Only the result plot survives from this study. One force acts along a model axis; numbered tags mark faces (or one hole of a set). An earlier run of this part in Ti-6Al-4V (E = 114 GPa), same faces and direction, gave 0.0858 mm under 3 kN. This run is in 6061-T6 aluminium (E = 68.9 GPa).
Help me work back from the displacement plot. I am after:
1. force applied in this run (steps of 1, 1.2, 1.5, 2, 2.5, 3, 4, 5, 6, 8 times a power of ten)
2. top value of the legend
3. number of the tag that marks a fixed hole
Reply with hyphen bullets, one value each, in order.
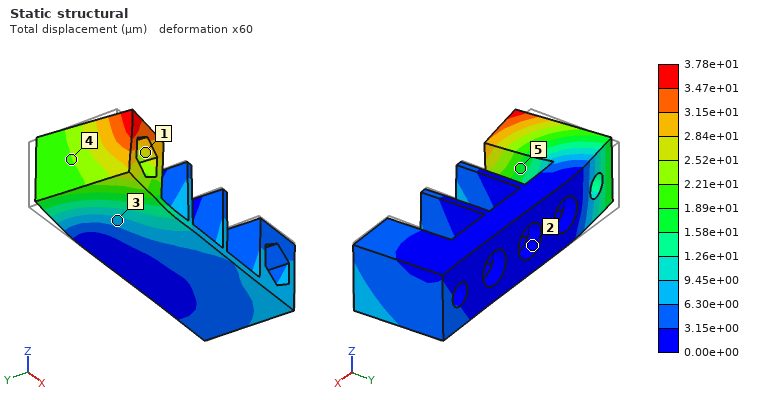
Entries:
- 800 N
- 3.78e+01 µm
- 2
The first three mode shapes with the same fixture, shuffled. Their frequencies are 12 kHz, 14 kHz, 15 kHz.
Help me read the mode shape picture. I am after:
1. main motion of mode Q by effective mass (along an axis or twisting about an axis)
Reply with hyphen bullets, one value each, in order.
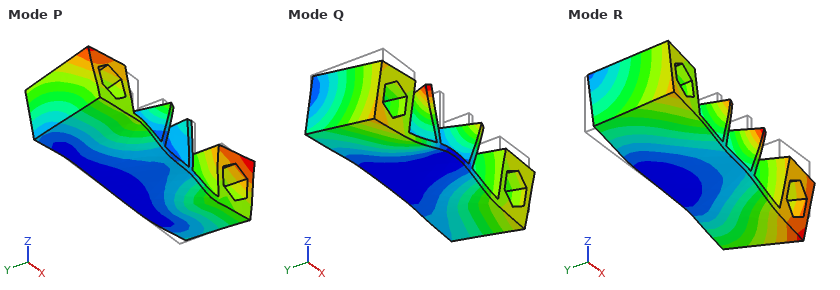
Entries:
- along Z
